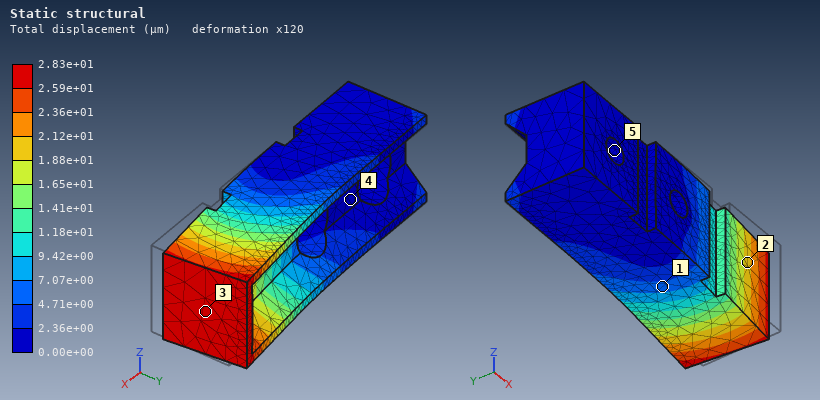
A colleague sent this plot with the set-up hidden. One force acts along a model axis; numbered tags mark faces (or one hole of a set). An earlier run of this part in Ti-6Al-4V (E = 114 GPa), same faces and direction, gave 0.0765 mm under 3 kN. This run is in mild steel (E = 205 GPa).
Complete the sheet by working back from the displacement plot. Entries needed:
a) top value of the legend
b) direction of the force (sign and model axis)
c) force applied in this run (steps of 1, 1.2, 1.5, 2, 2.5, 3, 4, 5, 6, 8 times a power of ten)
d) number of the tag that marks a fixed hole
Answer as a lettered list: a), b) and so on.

a) 2.83e+01 µm
b) +Y
c) 2 kN
d) 5
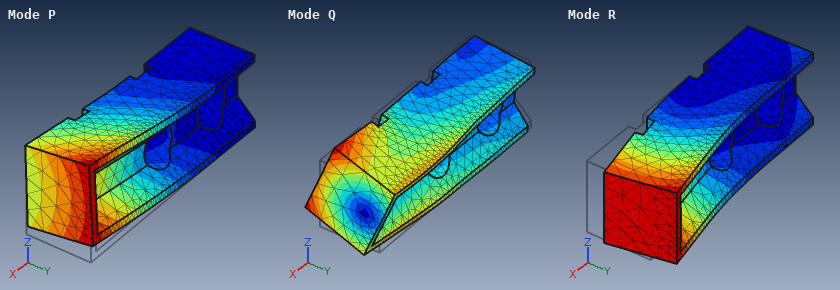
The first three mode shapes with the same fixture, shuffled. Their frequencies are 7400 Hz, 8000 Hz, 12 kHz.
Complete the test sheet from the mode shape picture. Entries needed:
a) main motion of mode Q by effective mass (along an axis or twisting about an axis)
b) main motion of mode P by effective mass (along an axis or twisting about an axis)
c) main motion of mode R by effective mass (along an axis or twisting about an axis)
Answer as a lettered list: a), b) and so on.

a) twisting about X
b) along Z
c) along Y
